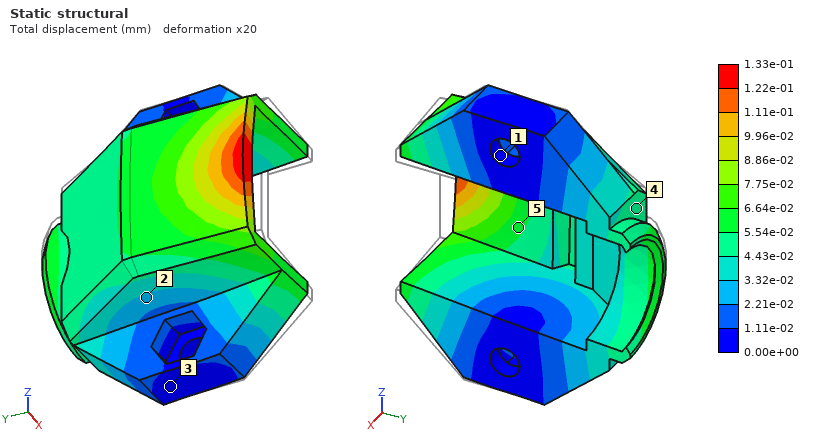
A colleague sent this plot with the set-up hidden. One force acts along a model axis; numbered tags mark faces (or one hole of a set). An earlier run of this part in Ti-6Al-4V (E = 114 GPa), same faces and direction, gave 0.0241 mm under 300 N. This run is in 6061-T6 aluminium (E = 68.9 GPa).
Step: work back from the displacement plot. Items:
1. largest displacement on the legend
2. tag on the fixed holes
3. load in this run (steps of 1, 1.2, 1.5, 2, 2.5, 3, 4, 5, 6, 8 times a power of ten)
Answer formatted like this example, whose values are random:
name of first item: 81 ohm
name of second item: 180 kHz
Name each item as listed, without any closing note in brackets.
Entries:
largest displacement on the legend: 1.33e-01 mm
tag on the fixed holes: 1
load in this run: 1 kN
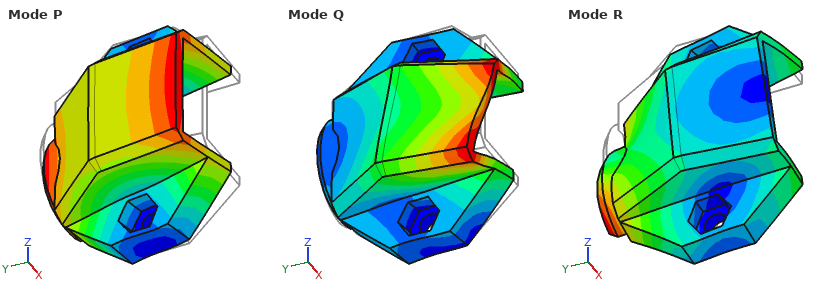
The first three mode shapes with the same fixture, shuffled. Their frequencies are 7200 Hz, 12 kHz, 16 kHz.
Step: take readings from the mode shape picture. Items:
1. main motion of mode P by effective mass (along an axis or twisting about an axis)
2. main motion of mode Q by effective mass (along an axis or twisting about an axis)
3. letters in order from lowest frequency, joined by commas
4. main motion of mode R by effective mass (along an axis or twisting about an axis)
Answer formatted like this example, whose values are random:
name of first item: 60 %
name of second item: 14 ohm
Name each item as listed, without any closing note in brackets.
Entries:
main motion of mode P by effective mass: along Y
main motion of mode Q by effective mass: along Z
letters in order from lowest frequency, joined by commas: P, Q, R
main motion of mode R by effective mass: along Z
